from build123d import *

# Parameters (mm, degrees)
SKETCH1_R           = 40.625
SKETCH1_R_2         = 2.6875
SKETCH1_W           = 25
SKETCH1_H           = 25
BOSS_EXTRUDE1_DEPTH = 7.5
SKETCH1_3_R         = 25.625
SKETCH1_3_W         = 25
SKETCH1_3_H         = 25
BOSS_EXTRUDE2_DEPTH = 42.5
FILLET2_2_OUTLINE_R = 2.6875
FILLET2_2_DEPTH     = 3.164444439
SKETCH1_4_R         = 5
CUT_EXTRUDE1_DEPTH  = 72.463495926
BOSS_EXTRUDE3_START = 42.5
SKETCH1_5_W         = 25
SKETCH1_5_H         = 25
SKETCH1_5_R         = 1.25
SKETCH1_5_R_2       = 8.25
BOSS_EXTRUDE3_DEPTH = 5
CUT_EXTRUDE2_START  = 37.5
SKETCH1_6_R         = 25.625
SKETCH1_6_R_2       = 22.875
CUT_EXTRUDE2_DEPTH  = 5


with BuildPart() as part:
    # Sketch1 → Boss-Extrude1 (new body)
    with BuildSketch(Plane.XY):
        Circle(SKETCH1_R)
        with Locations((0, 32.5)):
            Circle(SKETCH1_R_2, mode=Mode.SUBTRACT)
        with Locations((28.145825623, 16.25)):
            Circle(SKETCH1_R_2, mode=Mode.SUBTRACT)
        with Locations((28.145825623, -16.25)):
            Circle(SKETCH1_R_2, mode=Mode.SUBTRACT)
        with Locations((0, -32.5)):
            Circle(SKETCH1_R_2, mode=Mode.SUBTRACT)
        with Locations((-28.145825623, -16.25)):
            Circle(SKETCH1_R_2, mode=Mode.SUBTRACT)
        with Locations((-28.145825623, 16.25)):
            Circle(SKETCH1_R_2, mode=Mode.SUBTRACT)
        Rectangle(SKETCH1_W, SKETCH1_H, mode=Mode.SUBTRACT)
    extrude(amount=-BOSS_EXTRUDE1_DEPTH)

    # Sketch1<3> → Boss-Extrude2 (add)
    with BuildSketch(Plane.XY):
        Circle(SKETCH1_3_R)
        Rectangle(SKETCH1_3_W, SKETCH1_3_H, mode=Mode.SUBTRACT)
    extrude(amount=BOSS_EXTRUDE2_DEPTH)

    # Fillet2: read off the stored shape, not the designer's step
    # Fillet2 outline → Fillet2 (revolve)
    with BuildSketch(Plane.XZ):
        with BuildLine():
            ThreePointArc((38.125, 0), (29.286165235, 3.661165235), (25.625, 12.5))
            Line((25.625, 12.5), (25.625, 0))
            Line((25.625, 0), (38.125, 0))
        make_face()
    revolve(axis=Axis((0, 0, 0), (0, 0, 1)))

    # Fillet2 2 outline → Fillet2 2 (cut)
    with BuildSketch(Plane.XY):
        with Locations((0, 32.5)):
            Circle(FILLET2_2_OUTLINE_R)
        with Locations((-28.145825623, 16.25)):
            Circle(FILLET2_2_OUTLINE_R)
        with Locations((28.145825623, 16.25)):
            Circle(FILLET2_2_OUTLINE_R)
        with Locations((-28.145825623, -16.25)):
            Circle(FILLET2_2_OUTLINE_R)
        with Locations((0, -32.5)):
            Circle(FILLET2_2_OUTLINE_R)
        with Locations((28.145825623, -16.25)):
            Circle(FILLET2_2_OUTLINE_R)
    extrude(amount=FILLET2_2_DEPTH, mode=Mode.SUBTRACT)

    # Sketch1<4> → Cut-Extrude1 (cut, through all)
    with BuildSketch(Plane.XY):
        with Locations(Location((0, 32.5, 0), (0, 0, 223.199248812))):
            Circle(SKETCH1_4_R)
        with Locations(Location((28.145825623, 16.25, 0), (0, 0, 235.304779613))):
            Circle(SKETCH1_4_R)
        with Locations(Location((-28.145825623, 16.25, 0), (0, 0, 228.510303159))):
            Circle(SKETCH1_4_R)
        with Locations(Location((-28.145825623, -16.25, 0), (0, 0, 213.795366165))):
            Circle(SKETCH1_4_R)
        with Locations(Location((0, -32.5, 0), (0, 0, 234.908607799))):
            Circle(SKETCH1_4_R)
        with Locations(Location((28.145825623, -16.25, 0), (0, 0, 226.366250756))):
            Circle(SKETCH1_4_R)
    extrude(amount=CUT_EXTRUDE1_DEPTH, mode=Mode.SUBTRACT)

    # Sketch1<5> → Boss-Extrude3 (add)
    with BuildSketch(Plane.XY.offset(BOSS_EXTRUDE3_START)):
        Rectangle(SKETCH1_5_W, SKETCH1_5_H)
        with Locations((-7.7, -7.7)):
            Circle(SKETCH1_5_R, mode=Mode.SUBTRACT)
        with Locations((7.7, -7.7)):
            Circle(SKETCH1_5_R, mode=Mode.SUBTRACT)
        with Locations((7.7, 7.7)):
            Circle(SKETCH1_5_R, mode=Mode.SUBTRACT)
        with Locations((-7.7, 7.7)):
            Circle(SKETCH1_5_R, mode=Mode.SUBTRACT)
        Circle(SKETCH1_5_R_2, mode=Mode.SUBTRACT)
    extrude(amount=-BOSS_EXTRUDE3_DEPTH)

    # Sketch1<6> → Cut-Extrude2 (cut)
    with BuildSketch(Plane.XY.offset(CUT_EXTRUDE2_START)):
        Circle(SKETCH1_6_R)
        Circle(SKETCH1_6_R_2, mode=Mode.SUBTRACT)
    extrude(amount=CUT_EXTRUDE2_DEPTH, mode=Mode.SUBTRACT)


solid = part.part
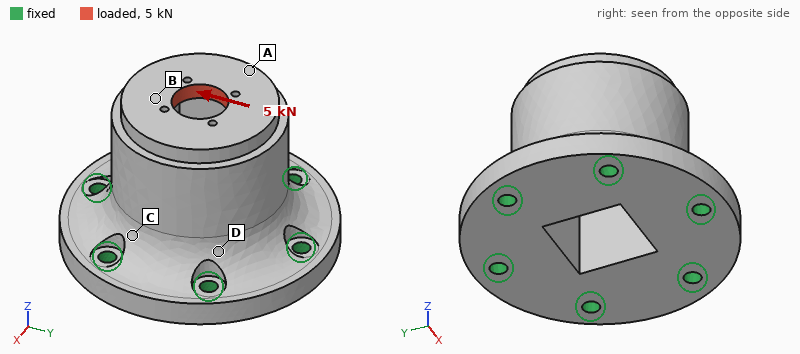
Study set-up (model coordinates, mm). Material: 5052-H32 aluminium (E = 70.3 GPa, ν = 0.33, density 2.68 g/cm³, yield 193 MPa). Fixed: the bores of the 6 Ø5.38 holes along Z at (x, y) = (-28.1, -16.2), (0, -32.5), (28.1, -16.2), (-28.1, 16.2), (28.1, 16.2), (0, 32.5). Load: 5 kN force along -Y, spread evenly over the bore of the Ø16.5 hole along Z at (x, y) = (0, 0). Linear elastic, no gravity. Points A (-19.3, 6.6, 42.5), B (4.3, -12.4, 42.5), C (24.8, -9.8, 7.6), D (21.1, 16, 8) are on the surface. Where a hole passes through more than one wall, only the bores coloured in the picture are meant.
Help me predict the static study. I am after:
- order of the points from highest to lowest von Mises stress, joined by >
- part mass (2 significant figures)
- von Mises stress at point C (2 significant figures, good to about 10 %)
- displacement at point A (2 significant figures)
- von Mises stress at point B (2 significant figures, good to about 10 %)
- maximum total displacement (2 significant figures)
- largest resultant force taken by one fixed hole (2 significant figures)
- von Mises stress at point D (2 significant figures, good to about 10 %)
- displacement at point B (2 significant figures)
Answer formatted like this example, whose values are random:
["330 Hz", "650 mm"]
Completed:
["B > D > C > A", "270 g", "11 MPa", "20 µm", "22 MPa", "26 µm", "2.6 kN", "16 MPa", "24 µm"]
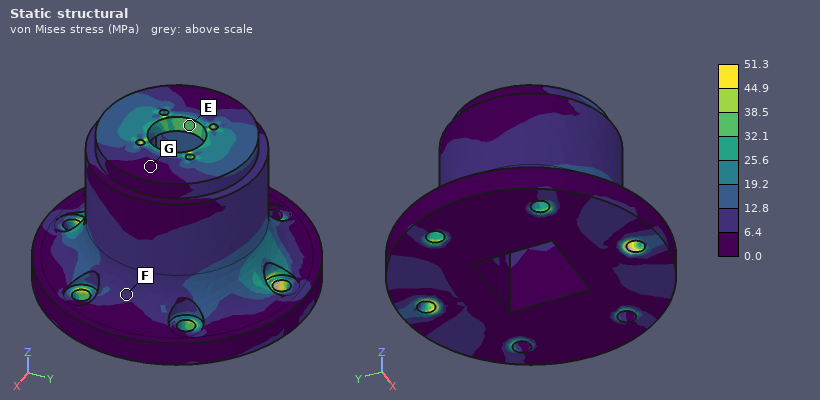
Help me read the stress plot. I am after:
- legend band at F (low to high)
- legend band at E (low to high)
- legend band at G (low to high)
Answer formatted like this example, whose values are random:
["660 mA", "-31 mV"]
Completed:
["6.4 to 12.8 MPa", "32.1 to 38.5 MPa", "0.0 to 6.4 MPa"]
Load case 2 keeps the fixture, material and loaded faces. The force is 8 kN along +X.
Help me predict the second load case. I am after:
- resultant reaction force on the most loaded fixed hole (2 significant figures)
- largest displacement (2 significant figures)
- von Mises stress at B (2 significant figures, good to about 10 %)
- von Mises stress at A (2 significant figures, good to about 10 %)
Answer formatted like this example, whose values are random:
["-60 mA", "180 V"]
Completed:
["3.7 kN", "42 µm", "12 MPa", "26 MPa"]
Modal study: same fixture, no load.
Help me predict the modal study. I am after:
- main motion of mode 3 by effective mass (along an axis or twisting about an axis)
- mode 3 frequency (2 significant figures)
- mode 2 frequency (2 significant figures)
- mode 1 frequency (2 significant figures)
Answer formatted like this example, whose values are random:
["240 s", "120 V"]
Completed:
["along Z", "15 kHz", "9800 Hz", "9800 Hz"]
